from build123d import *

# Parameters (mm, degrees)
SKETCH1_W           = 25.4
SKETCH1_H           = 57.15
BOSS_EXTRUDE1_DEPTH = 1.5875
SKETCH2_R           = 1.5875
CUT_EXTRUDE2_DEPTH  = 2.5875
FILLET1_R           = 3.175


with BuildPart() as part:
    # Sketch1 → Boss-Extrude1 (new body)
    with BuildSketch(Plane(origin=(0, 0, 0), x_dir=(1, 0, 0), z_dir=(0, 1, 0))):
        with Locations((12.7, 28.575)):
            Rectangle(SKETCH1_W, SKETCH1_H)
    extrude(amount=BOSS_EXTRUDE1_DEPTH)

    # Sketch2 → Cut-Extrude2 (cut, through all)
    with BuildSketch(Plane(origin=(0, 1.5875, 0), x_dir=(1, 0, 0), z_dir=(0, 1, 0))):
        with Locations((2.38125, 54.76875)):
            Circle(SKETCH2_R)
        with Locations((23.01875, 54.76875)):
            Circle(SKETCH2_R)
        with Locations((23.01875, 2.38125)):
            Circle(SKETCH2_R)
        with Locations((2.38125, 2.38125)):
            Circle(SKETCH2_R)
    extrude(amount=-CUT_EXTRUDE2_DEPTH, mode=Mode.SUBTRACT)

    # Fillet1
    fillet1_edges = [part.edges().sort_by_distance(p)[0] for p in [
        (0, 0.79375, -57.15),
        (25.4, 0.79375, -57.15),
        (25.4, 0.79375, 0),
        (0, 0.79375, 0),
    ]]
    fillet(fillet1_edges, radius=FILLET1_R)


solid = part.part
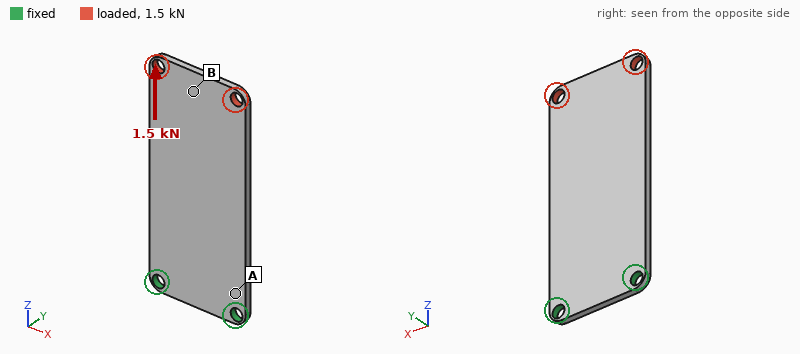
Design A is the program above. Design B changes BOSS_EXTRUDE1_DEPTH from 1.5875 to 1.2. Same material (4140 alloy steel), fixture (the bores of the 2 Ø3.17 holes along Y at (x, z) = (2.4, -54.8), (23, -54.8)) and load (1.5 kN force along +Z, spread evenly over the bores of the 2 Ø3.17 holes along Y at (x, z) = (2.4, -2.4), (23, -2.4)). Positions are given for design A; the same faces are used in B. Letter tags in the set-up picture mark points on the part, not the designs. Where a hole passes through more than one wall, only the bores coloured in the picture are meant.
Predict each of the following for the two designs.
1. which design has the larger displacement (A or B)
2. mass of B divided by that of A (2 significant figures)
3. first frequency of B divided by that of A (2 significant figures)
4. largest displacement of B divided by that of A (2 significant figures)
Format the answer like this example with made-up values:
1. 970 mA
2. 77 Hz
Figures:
1. B
2. 0.76
3. 0.76
4. 1.3
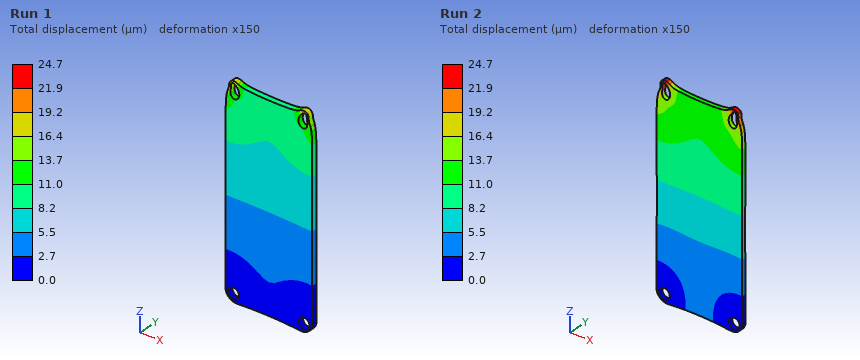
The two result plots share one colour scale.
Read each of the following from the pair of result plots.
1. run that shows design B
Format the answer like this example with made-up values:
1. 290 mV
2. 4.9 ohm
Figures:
1. Run 2
